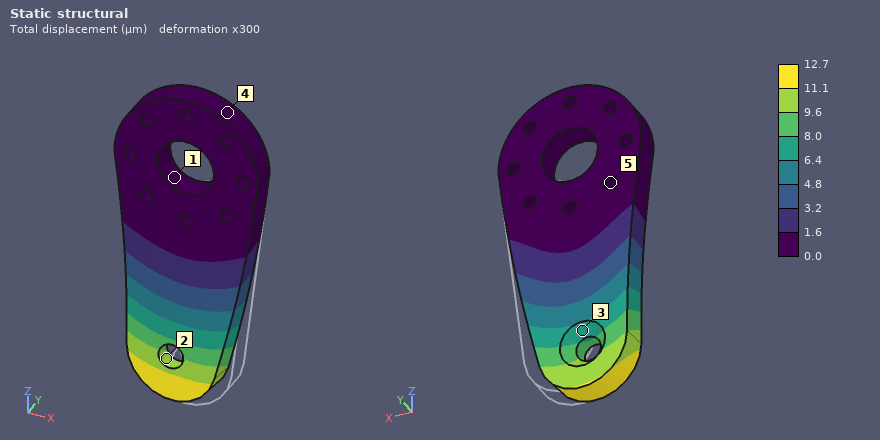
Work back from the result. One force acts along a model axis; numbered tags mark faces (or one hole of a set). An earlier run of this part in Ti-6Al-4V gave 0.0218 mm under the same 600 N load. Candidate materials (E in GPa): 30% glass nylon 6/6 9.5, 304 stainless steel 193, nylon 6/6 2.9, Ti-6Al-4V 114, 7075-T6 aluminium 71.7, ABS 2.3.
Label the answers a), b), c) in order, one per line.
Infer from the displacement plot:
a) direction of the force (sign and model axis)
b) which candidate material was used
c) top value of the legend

a) -X
b) 304 stainless steel
c) 12.7 µm
